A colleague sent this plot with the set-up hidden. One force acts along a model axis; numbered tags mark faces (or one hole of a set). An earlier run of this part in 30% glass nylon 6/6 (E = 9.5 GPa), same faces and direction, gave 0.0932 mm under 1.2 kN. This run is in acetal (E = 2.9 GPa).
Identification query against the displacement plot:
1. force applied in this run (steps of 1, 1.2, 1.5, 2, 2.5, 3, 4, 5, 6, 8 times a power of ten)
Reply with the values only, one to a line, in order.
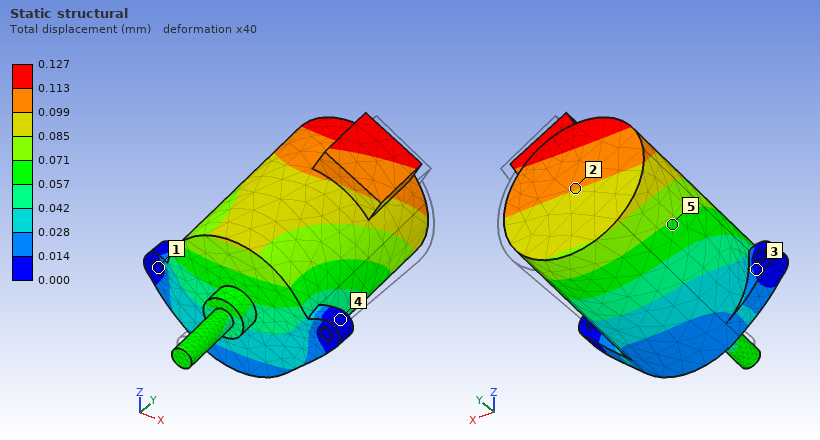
500 N
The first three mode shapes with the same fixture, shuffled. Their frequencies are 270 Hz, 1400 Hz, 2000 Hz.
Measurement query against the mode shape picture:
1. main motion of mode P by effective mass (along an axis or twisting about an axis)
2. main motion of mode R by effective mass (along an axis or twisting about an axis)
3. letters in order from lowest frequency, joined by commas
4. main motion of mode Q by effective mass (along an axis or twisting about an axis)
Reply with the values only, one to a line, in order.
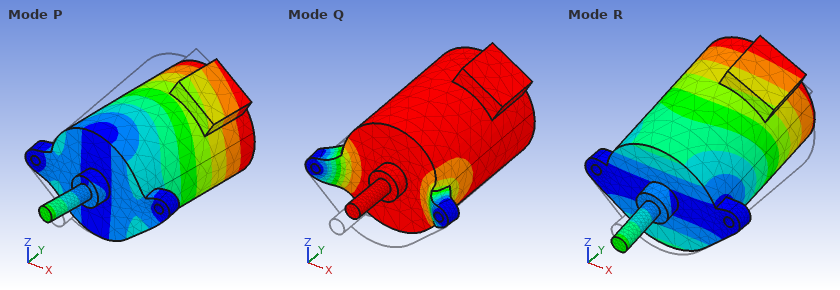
along X
along Z
R, P, Q
along Y
